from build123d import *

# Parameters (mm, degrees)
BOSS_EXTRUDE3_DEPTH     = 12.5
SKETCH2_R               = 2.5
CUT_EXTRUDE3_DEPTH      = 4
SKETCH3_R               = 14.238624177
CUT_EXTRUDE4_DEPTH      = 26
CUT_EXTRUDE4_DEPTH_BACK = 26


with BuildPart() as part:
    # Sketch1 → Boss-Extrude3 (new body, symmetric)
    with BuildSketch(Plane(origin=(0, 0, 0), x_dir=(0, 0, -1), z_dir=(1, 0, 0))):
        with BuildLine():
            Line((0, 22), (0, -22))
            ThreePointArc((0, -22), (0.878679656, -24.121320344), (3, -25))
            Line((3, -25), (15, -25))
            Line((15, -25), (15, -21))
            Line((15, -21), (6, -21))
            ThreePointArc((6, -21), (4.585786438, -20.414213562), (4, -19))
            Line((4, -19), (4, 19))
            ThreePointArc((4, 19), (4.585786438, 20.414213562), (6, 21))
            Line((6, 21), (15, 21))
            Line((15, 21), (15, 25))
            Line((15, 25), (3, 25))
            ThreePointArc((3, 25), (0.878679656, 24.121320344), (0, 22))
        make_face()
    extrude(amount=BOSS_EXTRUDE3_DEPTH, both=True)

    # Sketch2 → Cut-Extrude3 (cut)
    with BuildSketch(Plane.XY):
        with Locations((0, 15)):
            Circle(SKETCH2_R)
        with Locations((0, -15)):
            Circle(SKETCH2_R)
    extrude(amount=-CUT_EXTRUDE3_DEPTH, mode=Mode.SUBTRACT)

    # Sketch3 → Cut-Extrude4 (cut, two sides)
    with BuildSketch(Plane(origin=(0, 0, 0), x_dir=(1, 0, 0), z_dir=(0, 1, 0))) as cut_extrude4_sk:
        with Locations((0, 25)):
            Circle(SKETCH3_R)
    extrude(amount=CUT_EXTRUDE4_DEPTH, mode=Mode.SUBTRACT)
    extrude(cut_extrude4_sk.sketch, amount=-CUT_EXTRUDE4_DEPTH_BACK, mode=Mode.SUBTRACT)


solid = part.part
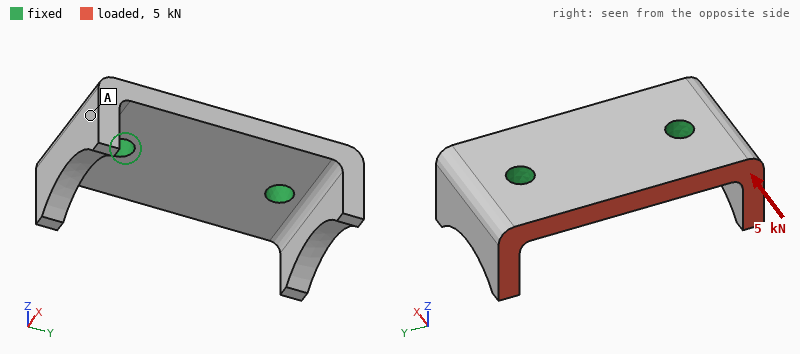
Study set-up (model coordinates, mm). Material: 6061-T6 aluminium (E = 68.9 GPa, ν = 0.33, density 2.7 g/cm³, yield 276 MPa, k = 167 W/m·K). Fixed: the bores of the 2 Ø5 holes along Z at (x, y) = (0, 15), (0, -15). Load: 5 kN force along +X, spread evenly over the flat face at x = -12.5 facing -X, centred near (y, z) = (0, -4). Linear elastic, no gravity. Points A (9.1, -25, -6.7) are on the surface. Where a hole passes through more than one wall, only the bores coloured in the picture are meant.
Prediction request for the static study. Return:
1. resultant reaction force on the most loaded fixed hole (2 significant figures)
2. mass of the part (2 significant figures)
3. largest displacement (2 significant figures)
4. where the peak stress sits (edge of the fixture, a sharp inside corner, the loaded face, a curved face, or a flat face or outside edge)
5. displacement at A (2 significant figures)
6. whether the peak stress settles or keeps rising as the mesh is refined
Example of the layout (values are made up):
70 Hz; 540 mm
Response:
2.5 kN; 18 g; 58 µm; edge of the fixture; 27 µm; keeps rising
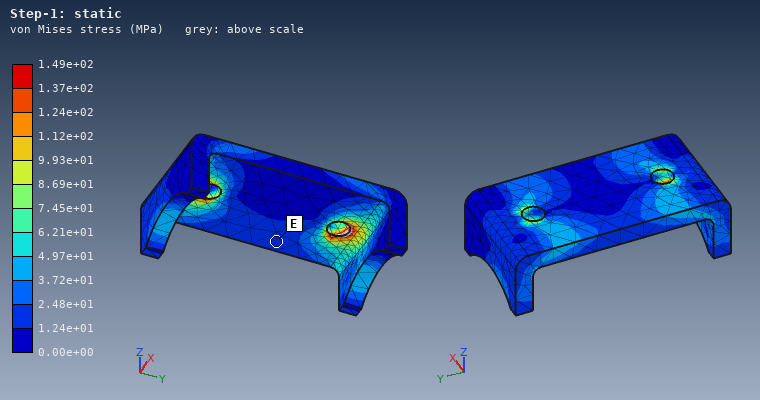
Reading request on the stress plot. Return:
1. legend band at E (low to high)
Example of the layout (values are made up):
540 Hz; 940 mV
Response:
1.24e+01 to 2.48e+01 MPa
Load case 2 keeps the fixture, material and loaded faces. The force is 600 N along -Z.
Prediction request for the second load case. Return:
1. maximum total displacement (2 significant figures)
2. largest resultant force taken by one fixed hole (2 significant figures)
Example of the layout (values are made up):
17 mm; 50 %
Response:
25 µm; 300 N
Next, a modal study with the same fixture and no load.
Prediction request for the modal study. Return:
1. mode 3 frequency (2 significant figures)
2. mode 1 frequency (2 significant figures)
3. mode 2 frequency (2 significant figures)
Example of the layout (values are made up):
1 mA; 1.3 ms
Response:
13 kHz; 12 kHz; 12 kHz
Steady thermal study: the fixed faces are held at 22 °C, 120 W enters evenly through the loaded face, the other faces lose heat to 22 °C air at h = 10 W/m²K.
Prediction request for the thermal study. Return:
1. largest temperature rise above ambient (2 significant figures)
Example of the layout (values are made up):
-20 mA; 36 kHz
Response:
55 K
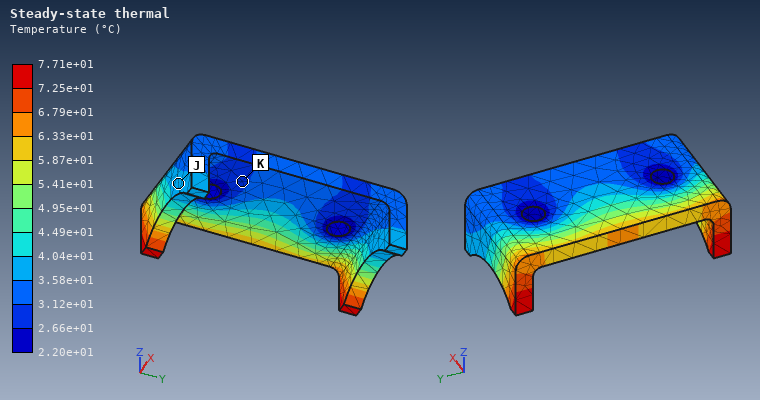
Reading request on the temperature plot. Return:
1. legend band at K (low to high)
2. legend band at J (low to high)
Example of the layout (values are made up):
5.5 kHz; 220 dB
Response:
2.66e+01 to 3.12e+01 °C; 3.58e+01 to 4.04e+01 °C
